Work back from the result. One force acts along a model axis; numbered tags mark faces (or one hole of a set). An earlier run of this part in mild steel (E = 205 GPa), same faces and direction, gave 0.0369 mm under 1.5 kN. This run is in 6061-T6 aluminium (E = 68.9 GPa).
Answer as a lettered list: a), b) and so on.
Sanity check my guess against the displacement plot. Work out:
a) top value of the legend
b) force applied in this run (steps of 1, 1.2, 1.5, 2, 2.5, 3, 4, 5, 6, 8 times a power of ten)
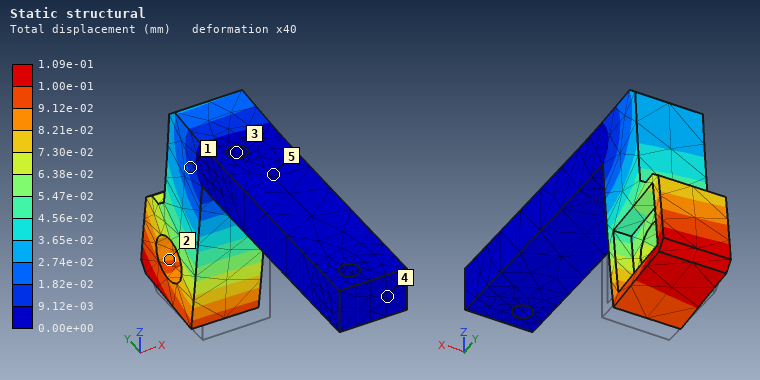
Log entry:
a) 1.09e-01 mm
b) 1.5 kN
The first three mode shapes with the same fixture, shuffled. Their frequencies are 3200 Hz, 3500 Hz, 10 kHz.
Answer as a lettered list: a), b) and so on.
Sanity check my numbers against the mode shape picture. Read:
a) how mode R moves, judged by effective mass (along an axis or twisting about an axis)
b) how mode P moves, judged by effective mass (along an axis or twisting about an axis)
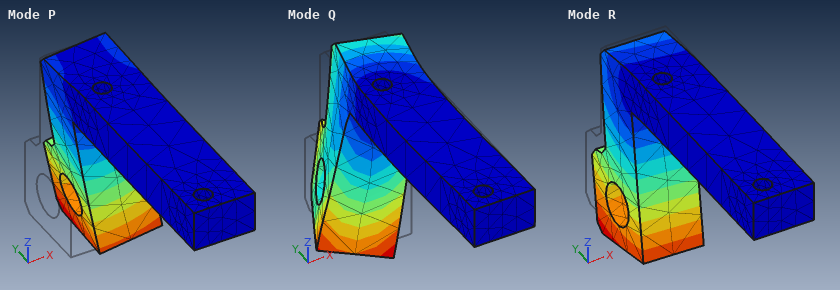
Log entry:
a) along Y
b) along X
